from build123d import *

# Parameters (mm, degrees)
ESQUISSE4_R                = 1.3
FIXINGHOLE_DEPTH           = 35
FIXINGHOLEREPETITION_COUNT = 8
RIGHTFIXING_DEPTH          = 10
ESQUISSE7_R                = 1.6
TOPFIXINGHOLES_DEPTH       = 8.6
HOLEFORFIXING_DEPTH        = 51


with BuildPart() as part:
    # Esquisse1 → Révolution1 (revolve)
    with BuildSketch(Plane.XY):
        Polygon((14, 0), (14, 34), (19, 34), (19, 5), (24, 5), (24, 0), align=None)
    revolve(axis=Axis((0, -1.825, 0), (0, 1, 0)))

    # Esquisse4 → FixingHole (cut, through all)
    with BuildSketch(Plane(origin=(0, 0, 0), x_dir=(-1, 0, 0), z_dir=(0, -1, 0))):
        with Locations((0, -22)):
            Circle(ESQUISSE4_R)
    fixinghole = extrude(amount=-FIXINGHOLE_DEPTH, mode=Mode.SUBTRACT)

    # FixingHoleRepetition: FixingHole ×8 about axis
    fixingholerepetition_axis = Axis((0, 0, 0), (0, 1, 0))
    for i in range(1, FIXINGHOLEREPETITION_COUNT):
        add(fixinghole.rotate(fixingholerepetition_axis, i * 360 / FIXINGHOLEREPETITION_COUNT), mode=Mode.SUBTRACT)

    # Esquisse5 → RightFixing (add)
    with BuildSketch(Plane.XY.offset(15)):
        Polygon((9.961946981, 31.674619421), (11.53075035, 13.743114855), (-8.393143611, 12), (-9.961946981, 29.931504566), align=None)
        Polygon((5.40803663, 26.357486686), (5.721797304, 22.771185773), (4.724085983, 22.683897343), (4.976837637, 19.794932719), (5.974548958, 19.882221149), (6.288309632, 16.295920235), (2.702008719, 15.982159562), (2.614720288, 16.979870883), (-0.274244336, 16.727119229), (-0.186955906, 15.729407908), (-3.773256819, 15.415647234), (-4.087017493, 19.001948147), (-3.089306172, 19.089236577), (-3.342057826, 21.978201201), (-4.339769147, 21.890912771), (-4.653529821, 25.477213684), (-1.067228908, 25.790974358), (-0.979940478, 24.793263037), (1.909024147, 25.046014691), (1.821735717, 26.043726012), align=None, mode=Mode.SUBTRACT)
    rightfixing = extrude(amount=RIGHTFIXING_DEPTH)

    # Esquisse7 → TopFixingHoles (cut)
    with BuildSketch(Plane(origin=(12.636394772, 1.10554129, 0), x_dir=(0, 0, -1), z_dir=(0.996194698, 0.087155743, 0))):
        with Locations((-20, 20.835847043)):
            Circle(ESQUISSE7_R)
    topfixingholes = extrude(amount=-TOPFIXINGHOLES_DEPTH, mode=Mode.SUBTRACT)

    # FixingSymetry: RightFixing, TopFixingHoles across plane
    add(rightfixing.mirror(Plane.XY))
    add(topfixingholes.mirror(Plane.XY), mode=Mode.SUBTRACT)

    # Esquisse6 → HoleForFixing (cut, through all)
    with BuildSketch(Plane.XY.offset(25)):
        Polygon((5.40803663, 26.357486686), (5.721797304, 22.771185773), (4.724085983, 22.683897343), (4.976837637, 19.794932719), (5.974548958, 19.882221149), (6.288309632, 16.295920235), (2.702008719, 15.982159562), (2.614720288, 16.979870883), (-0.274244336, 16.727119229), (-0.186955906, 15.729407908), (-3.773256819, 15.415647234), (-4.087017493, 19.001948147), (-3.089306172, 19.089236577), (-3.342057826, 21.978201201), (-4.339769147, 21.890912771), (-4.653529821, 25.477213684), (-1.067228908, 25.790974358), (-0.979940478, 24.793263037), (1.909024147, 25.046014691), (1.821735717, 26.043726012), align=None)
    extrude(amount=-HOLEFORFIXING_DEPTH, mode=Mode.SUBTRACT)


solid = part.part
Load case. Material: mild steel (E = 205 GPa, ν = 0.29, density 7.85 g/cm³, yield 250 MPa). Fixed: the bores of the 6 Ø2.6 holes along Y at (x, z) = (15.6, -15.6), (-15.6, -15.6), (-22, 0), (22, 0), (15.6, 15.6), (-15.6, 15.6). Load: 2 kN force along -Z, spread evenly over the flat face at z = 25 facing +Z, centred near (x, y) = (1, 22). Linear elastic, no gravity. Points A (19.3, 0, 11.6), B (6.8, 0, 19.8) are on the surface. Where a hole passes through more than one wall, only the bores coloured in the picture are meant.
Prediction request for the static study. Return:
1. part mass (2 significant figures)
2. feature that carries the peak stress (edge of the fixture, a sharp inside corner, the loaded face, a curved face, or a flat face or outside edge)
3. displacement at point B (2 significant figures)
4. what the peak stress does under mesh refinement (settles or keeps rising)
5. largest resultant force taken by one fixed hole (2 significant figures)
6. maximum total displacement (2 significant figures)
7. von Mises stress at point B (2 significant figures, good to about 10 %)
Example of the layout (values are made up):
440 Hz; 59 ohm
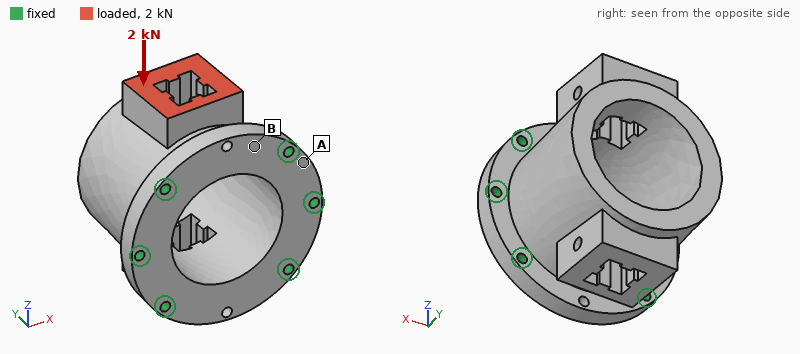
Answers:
190 g; edge of the fixture; 2.6 µm; keeps rising; 860 N; 10 µm; 16 MPa
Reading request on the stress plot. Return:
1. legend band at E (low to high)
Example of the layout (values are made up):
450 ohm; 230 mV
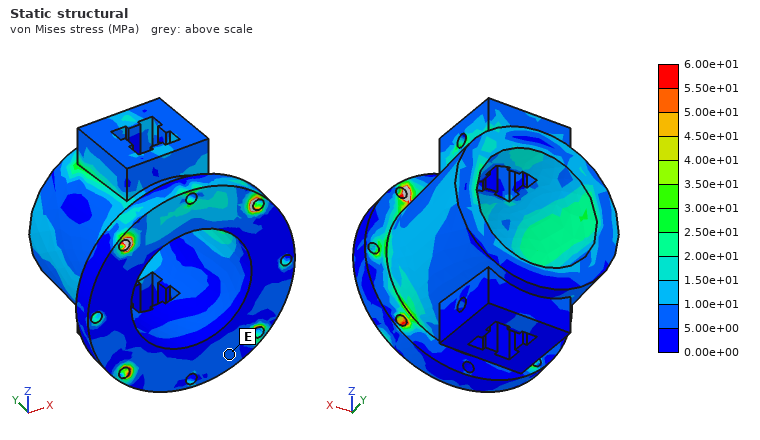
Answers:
5.00e+00 to 1.00e+01 MPa
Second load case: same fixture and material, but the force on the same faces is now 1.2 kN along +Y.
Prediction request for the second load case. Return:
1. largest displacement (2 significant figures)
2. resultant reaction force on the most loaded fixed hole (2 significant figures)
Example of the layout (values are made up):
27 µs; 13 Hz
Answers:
9.3 µm; 800 N
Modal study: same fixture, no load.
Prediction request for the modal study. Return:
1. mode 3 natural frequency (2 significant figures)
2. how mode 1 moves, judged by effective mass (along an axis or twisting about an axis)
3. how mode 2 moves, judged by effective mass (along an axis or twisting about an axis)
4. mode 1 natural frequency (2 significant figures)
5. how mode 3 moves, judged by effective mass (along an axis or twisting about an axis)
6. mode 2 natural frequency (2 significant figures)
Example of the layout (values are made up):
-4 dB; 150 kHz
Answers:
13 kHz; along Z; along X; 8800 Hz; along Y; 11 kHz
